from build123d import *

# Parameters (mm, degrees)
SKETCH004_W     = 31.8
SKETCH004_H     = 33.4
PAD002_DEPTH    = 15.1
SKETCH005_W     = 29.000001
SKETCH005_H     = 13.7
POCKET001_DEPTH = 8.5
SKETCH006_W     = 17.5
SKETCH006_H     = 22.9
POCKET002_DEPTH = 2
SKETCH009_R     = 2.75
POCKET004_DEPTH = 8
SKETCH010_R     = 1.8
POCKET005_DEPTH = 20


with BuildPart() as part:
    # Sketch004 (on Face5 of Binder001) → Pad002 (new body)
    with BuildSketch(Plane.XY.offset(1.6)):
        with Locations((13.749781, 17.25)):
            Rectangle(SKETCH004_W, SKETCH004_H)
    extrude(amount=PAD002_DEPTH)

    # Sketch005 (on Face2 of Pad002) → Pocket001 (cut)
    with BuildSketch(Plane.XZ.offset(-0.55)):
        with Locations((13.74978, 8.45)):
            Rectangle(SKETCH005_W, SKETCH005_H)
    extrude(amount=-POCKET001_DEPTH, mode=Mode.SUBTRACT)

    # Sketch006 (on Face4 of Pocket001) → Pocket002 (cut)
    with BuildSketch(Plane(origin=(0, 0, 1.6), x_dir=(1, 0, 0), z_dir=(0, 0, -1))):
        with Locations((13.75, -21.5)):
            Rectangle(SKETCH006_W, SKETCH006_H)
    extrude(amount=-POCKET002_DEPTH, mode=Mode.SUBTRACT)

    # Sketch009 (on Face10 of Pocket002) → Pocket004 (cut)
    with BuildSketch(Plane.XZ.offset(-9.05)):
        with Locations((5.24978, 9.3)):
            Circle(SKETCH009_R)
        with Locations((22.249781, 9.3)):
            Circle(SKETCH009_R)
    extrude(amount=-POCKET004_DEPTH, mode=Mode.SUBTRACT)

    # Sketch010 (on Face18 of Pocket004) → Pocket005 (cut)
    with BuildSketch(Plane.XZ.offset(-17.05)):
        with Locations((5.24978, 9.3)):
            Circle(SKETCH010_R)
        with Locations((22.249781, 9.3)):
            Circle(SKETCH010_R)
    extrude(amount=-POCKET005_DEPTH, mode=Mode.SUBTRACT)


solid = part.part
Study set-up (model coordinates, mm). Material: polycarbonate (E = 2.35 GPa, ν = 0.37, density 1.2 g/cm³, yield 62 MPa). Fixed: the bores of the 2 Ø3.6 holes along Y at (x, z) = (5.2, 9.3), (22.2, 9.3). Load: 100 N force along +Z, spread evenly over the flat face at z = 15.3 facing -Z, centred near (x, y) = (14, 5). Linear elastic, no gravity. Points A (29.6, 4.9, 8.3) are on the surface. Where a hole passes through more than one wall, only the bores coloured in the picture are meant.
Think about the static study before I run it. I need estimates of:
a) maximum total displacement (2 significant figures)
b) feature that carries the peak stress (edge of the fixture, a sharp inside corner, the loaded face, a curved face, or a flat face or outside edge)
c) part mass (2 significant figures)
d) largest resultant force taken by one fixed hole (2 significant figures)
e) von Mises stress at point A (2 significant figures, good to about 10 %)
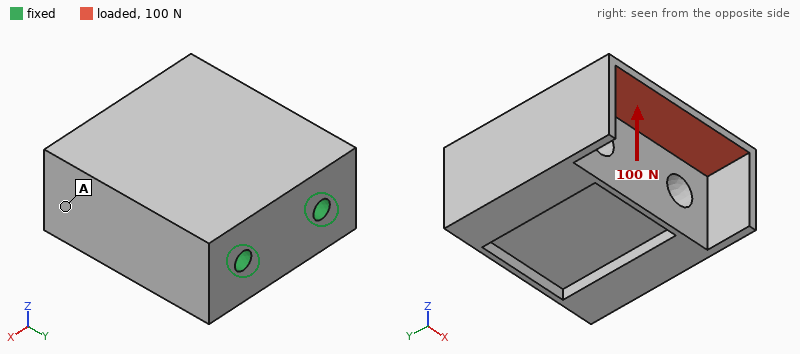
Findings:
0.50 mm
a flat face or outside edge
13 g
50 N
2.2 MPa
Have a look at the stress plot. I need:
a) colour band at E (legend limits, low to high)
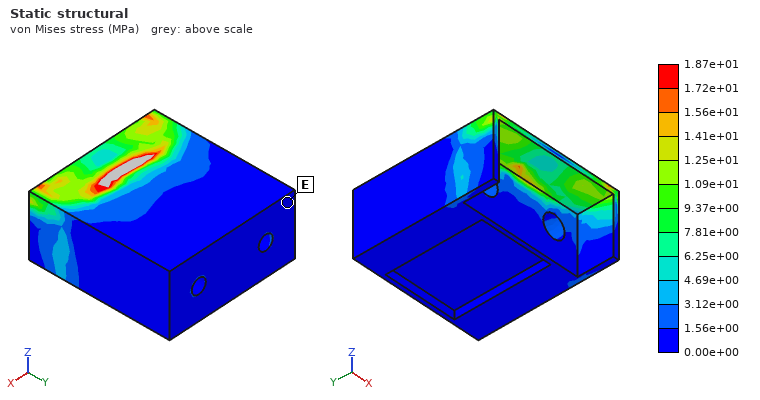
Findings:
0.00e+00 to 1.56e+00 MPa
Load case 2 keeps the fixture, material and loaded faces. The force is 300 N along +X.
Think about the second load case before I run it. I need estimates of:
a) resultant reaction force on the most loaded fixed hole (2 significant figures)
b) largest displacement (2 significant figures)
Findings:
270 N
0.11 mm
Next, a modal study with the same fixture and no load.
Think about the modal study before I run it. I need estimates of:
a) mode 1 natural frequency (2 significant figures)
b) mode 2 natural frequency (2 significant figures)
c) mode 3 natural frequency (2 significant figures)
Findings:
4500 Hz
4800 Hz
5100 Hz
